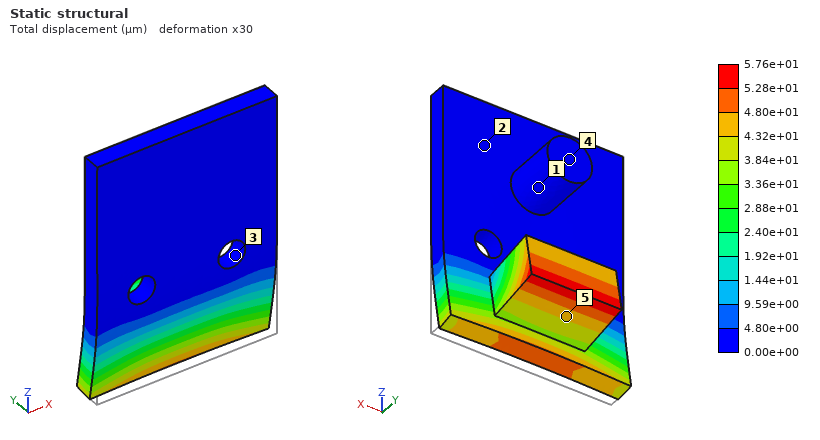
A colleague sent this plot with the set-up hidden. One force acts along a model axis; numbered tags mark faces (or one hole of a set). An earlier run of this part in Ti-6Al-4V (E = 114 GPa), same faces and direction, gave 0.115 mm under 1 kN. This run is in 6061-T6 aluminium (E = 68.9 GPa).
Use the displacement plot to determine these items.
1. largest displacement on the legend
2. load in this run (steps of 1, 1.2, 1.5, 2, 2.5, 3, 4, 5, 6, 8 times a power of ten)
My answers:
5.76e+01 µm
300 N
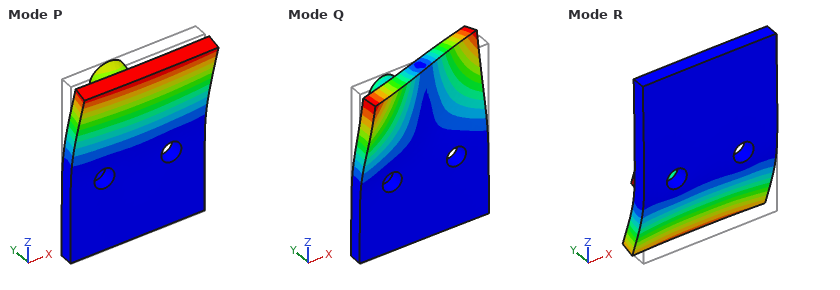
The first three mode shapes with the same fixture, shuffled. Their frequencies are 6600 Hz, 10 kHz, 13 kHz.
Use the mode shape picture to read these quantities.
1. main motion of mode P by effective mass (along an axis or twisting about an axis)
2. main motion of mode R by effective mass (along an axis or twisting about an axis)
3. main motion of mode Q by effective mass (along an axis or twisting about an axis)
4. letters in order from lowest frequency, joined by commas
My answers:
along Y
along Y
twisting about Z
P, R, Q
